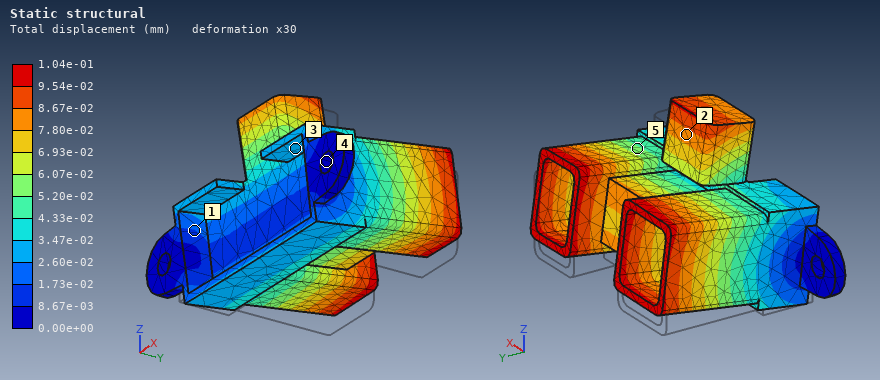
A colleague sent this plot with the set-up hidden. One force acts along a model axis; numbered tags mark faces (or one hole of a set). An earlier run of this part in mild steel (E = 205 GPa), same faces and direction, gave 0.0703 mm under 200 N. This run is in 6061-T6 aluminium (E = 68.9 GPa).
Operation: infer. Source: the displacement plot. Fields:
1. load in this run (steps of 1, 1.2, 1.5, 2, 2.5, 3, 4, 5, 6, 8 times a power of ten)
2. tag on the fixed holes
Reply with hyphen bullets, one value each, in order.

- 100 N
- 4
